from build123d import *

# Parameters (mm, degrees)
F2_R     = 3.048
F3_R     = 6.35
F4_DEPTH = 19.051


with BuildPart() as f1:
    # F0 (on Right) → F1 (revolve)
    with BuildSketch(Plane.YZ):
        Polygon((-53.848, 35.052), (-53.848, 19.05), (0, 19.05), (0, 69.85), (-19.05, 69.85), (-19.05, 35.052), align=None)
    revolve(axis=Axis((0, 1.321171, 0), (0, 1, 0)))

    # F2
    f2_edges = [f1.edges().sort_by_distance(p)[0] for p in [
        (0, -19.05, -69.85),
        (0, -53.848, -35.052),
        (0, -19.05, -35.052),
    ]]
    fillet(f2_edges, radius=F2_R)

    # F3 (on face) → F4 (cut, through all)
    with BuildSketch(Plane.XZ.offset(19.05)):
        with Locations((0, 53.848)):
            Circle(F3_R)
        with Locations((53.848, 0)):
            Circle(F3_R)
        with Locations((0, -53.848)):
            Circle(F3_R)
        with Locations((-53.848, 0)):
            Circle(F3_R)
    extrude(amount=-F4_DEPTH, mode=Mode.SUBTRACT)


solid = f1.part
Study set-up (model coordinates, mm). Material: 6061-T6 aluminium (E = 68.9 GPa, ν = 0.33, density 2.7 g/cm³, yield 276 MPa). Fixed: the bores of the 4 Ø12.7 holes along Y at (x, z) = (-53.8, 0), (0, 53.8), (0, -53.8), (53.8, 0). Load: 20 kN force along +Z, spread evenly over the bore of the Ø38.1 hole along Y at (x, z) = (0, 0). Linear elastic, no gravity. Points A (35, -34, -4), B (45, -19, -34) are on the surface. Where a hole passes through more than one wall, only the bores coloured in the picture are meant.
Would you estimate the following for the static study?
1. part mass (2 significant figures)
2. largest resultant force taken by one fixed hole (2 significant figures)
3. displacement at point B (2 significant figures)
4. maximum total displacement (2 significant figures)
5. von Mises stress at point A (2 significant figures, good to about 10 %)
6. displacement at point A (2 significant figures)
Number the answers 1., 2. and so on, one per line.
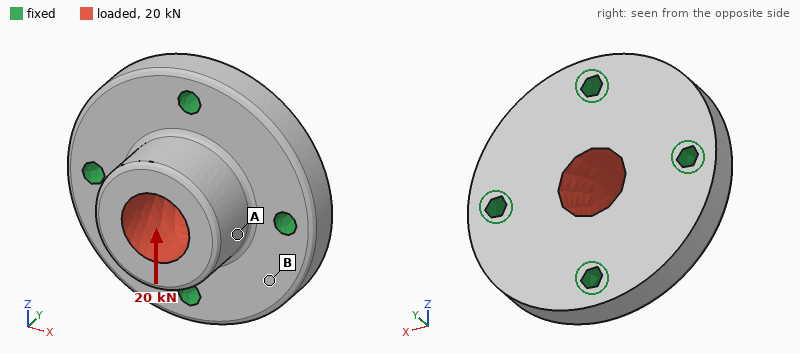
1. 960 g
2. 7.2 kN
3. 3.4 µm
4. 17 µm
5. 5.4 MPa
6. 8.7 µm
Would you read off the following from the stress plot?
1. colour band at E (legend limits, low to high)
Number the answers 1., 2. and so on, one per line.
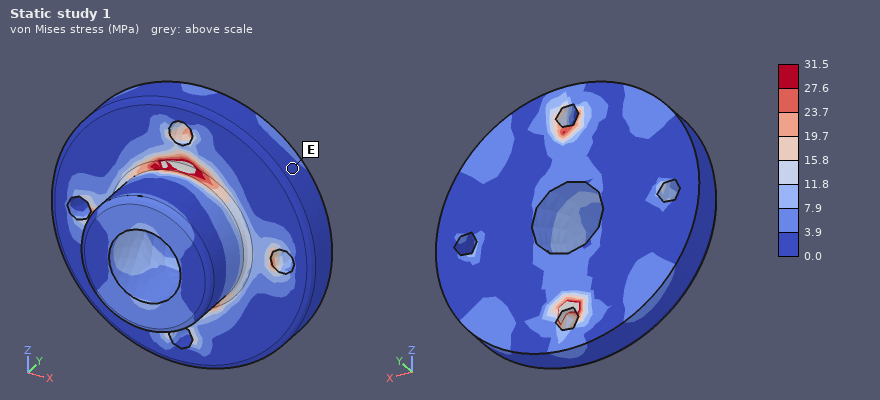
1. 0.0 to 3.9 MPa
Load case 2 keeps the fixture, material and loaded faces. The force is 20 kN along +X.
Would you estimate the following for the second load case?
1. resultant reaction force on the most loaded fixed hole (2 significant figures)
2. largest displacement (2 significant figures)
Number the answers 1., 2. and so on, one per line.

1. 7.2 kN
2. 17 µm
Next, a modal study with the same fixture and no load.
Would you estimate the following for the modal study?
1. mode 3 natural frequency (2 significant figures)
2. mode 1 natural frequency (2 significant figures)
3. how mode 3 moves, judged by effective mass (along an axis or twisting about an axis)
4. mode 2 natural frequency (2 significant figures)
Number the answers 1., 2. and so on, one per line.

1. 9700 Hz
2. 9200 Hz
3. along Y
4. 9200 Hz
